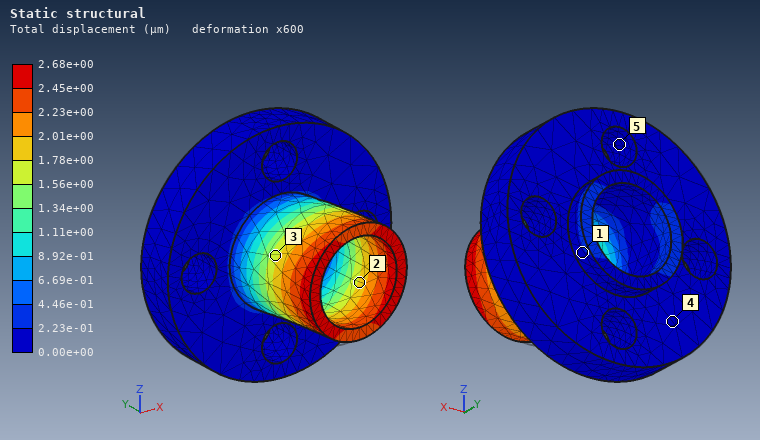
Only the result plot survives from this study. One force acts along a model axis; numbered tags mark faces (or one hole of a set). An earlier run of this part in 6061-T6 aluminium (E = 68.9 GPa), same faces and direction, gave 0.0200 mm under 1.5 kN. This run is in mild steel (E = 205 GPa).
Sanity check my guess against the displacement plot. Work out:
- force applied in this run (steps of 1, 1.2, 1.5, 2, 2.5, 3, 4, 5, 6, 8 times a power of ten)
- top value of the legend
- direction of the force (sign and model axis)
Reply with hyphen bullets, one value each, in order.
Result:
- 600 N
- 2.68e+00 µm
- +X
